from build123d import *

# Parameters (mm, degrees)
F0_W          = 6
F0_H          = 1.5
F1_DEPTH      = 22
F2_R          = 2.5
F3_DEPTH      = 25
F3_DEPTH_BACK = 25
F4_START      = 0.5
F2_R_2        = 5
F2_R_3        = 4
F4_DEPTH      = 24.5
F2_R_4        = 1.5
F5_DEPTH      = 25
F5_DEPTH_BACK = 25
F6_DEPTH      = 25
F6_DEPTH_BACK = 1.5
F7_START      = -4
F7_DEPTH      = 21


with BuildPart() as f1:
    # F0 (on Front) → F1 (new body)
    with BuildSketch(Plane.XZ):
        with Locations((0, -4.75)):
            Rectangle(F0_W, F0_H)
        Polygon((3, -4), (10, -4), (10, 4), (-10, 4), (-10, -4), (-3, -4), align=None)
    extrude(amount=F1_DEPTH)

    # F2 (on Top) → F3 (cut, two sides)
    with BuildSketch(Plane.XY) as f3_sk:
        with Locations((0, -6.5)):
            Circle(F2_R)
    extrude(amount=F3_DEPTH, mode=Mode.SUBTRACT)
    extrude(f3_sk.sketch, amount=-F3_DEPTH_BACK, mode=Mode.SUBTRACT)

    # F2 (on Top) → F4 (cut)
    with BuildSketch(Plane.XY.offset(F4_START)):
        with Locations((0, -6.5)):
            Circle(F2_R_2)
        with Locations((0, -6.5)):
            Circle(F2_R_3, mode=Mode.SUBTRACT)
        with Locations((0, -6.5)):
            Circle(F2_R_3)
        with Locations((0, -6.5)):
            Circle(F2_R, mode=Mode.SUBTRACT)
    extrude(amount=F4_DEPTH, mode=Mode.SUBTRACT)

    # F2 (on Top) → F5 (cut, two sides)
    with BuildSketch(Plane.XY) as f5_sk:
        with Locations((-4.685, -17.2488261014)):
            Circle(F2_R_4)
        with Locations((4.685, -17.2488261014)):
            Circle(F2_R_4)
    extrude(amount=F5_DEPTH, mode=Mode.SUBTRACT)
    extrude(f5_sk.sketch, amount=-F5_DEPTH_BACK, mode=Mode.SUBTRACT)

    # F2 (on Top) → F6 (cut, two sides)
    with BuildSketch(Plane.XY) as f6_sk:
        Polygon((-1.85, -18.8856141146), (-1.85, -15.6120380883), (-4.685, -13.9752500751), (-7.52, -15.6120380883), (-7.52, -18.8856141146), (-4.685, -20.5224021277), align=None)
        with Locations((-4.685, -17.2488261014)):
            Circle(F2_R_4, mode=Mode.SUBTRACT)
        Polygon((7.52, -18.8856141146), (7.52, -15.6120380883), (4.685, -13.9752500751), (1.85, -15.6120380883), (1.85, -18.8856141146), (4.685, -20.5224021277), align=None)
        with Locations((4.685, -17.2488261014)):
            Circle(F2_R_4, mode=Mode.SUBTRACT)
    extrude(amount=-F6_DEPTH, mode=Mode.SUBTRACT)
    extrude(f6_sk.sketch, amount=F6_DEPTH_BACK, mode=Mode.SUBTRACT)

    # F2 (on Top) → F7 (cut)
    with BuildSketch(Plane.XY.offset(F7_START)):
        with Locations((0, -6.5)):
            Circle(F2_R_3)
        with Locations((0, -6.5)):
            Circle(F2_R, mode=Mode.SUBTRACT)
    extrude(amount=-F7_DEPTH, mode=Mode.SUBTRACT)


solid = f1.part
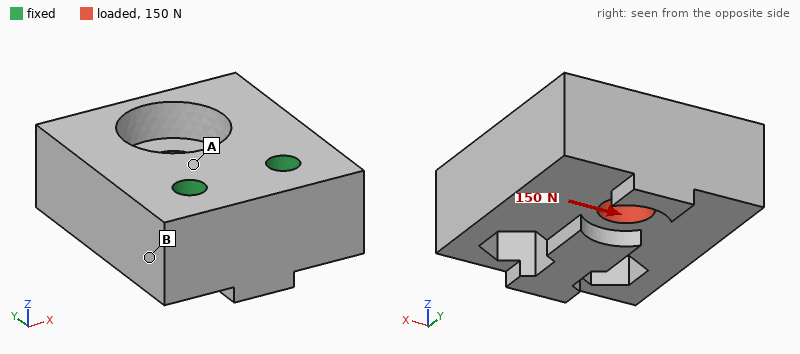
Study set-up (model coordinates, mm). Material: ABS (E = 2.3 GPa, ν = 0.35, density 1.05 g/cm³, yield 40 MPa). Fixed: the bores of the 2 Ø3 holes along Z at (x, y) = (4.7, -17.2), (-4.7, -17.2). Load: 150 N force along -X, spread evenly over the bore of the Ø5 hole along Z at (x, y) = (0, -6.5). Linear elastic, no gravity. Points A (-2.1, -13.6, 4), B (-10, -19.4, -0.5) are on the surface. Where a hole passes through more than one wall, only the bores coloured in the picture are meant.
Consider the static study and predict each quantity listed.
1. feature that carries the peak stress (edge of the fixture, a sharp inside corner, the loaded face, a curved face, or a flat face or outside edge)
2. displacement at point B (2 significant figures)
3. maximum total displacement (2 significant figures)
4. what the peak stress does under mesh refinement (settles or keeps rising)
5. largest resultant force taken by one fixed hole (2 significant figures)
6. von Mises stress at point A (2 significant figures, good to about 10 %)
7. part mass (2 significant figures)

edge of the fixture
31 µm
95 µm
keeps rising
160 N
5.8 MPa
3.1 g
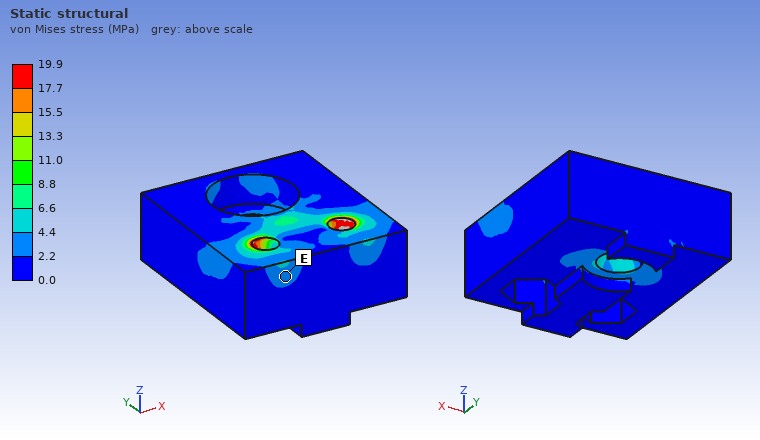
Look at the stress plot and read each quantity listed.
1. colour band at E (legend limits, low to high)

2.2 to 4.4 MPa
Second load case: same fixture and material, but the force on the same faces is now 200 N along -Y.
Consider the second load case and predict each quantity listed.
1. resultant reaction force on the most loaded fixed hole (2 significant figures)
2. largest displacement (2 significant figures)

100 N
0.26 mm
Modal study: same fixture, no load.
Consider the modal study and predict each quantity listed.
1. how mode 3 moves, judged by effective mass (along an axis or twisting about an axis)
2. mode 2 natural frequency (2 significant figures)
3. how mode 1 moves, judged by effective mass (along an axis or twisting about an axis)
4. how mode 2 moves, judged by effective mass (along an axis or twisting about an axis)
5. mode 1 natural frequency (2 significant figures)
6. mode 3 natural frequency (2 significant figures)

along X
5000 Hz
along Z
along X
2400 Hz
6100 Hz
